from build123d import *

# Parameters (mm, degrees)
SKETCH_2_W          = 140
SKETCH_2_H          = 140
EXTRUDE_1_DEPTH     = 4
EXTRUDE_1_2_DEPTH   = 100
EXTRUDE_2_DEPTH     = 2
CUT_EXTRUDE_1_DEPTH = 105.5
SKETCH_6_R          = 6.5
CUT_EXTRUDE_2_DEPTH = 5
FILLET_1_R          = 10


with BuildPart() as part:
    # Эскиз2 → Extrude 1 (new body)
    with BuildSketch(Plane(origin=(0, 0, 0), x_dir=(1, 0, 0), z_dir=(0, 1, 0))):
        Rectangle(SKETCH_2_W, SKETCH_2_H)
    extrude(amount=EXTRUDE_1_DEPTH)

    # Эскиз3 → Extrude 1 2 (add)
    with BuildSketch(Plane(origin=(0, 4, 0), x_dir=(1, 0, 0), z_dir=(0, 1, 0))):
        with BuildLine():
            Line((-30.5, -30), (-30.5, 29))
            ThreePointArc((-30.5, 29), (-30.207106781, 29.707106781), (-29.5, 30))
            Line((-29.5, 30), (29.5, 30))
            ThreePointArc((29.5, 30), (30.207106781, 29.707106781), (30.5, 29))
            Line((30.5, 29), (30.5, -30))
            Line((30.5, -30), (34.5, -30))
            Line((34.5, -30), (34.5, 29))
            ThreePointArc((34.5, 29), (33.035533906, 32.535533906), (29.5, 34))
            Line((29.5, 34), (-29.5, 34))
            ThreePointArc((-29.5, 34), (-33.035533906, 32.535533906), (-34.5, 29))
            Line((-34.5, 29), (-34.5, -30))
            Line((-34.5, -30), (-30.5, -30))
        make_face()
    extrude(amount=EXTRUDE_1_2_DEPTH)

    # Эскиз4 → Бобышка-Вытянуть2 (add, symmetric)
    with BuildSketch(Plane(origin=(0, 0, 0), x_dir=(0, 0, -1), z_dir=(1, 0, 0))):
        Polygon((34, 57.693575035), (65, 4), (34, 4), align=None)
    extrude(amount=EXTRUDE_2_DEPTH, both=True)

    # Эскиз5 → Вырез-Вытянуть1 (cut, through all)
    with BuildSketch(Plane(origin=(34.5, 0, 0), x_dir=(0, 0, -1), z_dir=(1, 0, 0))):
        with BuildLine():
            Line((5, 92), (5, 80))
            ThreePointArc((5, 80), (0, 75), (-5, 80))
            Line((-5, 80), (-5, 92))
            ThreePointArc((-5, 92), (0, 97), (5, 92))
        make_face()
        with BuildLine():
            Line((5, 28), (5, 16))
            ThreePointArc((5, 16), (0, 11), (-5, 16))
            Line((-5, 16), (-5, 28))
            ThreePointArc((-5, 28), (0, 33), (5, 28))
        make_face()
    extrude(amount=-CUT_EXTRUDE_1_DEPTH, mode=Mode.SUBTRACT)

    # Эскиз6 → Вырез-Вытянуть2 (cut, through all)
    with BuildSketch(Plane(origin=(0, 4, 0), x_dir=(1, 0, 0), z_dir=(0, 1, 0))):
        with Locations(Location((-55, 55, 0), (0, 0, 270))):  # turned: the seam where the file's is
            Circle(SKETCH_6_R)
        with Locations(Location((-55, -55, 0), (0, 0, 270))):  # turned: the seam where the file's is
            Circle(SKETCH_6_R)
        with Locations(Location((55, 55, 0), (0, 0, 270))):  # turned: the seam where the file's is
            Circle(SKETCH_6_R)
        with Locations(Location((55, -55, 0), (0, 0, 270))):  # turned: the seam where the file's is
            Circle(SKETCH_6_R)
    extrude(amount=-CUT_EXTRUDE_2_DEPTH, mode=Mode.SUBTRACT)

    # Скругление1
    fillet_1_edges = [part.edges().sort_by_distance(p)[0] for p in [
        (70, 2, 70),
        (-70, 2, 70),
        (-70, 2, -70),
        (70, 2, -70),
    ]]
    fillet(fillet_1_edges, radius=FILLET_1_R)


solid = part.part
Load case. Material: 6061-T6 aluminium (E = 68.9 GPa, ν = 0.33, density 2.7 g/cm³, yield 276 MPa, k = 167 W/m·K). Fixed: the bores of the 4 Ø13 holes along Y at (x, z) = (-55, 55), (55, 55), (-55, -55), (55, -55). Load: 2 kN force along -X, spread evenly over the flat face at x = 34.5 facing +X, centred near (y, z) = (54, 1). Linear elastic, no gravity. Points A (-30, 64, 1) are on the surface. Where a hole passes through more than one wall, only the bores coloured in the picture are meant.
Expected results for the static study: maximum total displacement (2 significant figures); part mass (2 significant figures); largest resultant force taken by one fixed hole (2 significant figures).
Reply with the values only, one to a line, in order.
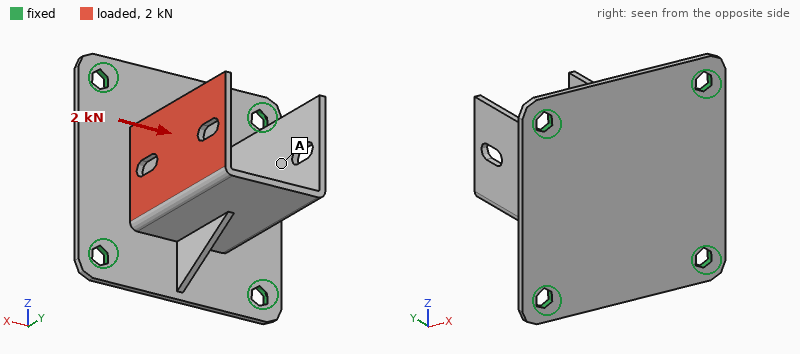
2.6 mm
410 g
1.2 kN
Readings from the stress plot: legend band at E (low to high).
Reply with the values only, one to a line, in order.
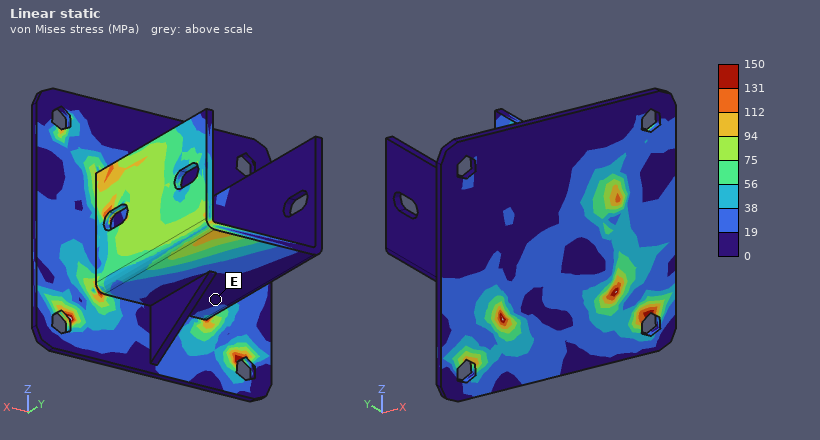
0 to 19 MPa
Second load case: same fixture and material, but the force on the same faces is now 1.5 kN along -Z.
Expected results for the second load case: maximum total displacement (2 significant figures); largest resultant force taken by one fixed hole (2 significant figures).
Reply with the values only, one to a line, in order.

0.56 mm
920 N
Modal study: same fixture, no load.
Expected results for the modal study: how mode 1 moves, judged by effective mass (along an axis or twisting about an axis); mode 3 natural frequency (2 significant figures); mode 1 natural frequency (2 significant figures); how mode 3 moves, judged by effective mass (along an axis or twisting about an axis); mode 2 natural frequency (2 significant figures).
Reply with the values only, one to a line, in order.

along X
1000 Hz
680 Hz
along Z
860 Hz
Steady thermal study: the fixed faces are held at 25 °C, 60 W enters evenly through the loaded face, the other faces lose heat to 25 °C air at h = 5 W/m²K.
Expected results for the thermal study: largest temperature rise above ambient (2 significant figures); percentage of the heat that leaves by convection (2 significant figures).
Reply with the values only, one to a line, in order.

65 K
11 %
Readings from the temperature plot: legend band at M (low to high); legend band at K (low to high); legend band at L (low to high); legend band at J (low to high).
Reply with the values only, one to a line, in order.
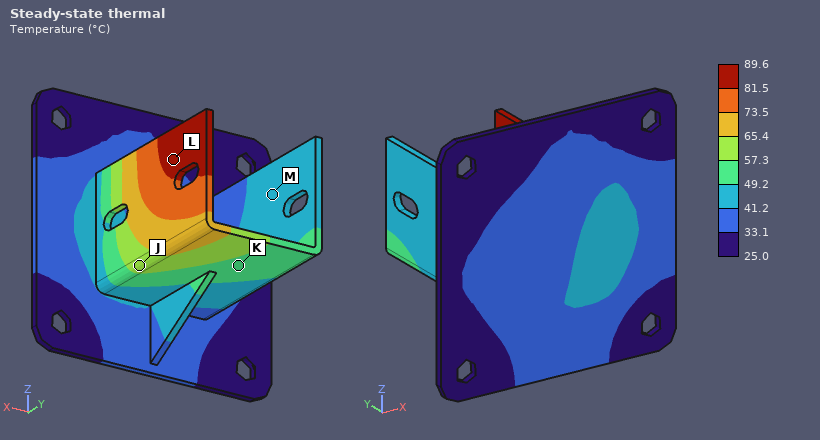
41.2 to 49.2 °C
49.2 to 57.3 °C
81.5 to 89.6 °C
57.3 to 65.4 °C
